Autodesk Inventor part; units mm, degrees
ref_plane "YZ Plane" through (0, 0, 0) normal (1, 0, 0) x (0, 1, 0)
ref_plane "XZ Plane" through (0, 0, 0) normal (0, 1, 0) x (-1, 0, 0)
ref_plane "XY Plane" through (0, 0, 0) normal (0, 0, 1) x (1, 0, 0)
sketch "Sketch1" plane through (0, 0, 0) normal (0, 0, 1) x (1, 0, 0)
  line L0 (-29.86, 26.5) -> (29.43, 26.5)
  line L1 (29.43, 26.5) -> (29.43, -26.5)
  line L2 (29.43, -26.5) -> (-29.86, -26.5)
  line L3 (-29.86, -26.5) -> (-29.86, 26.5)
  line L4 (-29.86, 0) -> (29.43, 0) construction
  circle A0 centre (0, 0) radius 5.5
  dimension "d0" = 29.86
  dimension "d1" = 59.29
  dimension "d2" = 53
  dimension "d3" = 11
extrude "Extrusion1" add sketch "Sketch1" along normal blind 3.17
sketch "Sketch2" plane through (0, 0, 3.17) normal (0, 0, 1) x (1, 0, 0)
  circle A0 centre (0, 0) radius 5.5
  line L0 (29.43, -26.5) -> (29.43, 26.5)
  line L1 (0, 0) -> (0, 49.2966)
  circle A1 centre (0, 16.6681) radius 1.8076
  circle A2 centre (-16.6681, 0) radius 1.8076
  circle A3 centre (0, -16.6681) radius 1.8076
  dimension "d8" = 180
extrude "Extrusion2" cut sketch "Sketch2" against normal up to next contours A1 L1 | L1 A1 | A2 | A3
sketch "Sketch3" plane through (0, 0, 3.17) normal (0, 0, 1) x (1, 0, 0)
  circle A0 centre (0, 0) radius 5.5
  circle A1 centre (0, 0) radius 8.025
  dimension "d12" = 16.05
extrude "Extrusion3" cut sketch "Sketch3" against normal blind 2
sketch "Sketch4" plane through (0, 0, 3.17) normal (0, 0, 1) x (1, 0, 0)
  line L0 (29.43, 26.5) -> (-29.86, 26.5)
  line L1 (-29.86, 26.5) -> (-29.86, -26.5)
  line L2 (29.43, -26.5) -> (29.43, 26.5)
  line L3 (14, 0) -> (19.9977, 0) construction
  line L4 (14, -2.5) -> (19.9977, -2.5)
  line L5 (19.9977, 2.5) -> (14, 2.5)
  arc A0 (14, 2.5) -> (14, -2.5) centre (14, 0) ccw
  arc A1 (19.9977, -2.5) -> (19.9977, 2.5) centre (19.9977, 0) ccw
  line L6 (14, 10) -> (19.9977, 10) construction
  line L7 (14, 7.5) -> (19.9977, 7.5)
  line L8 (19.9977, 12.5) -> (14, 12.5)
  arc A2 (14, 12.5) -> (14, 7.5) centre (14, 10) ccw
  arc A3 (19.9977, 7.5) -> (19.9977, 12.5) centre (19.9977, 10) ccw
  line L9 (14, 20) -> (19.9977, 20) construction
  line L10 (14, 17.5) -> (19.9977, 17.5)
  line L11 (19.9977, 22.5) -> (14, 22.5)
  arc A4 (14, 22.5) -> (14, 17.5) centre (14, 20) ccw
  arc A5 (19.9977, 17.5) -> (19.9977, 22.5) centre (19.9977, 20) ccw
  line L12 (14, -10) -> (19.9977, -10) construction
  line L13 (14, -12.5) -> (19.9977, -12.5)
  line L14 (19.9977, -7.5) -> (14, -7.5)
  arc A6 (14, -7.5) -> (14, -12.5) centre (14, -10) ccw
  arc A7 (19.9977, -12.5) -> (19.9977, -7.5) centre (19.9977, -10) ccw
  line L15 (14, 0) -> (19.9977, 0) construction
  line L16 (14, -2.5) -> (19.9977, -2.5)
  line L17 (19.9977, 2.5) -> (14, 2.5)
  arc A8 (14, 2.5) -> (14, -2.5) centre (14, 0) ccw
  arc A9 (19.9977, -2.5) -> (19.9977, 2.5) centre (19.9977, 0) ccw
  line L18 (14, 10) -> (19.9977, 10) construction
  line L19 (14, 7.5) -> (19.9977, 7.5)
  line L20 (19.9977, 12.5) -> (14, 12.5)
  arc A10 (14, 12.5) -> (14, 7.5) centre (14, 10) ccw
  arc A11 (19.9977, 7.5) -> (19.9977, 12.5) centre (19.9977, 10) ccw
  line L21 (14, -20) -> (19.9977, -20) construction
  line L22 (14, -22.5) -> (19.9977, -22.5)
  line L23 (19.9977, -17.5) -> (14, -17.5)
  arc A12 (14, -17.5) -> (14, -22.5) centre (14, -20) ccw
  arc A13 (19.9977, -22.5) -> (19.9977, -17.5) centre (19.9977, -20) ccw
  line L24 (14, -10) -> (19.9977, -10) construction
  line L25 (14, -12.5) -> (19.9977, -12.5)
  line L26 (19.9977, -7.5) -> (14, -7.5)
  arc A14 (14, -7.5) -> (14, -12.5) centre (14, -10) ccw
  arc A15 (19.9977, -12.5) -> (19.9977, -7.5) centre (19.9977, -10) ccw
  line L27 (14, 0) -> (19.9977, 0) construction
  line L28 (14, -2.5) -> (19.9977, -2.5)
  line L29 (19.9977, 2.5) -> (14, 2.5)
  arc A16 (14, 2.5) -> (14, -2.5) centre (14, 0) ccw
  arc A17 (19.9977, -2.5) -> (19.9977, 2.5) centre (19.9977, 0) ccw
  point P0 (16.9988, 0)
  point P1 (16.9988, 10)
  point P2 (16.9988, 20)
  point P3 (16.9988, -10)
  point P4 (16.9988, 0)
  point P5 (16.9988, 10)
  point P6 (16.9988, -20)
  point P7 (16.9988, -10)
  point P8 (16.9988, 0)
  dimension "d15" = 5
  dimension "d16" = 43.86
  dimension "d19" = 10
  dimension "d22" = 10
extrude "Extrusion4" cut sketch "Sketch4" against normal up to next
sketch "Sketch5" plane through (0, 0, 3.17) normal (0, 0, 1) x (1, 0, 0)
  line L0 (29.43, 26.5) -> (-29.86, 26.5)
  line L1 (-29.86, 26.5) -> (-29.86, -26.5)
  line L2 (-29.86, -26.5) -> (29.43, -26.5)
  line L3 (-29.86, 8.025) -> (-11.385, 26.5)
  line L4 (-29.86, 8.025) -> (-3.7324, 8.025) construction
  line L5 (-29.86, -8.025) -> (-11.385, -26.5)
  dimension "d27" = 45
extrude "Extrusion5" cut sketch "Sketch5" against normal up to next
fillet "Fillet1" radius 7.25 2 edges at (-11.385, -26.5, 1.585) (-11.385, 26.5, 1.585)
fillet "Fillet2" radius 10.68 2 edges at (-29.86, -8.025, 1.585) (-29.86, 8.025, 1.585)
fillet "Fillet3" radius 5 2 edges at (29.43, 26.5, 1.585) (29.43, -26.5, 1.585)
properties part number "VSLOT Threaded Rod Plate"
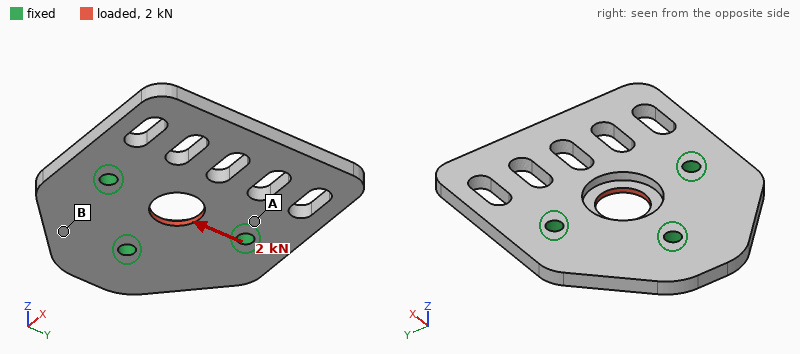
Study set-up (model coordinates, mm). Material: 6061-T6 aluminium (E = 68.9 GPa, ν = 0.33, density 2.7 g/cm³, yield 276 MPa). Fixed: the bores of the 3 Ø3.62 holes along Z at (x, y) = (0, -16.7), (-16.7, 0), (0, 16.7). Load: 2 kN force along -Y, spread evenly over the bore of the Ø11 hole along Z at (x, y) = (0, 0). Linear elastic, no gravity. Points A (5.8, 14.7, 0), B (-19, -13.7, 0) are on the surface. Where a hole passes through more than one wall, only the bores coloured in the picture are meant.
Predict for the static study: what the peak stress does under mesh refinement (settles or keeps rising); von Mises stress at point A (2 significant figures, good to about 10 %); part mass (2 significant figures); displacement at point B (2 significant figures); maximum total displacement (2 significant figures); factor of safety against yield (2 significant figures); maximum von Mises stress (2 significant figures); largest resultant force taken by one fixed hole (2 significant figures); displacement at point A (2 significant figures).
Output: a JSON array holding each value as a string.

["settles", "13 MPa", "20 g", "1.8 µm", "9.3 µm", "3.1", "90 MPa", "850 N", "2.5 µm"]
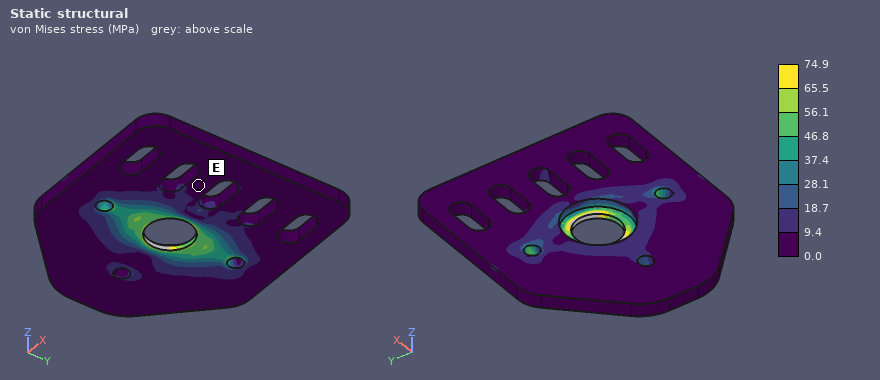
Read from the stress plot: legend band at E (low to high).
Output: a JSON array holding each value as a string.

["0.0 to 9.4 MPa"]
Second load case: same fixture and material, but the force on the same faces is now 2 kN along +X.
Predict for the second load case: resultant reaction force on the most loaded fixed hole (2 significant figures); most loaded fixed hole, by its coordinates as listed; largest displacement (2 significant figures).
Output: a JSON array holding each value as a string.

["750 N", "(-16.7, 0)", "30 µm"]
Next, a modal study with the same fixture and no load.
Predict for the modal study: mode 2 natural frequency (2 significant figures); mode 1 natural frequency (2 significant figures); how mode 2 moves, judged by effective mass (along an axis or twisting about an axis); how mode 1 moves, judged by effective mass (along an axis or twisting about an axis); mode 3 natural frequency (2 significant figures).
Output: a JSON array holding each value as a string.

["4600 Hz", "2700 Hz", "twisting about X", "along Z", "8100 Hz"]
